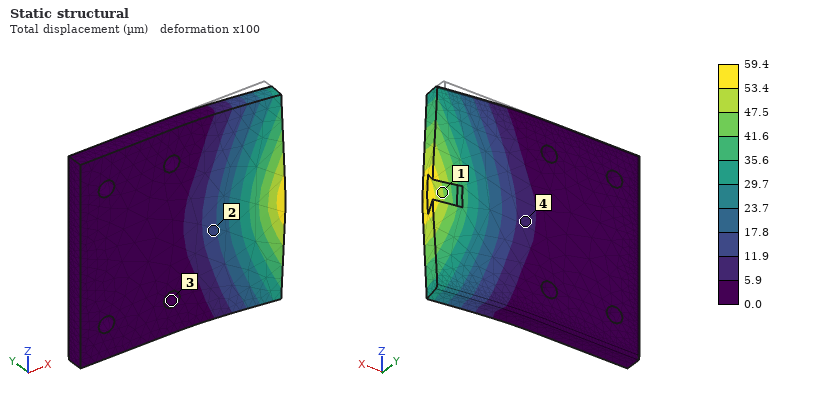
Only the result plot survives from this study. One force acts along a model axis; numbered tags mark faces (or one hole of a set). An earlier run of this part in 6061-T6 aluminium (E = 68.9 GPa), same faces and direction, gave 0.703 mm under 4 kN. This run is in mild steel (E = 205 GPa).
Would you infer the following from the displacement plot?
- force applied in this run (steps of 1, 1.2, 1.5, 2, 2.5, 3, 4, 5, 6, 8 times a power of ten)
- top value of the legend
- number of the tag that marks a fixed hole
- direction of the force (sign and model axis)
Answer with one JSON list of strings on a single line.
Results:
["1 kN", "59.4 µm", "3", "-Y"]
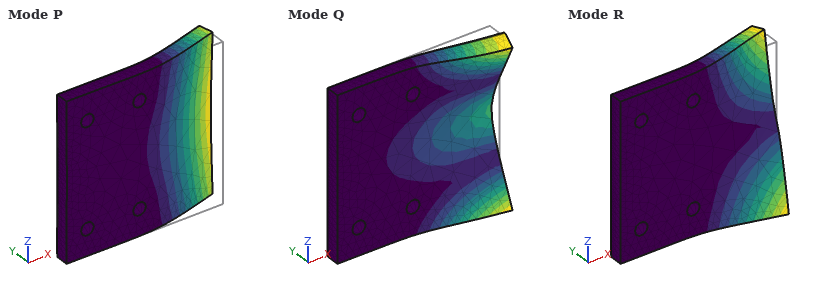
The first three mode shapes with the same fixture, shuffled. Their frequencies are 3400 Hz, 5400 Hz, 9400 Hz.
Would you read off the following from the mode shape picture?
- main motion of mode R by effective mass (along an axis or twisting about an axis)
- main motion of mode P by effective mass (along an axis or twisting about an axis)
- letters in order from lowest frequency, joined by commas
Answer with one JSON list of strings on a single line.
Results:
["twisting about X", "along Y", "P, R, Q"]
